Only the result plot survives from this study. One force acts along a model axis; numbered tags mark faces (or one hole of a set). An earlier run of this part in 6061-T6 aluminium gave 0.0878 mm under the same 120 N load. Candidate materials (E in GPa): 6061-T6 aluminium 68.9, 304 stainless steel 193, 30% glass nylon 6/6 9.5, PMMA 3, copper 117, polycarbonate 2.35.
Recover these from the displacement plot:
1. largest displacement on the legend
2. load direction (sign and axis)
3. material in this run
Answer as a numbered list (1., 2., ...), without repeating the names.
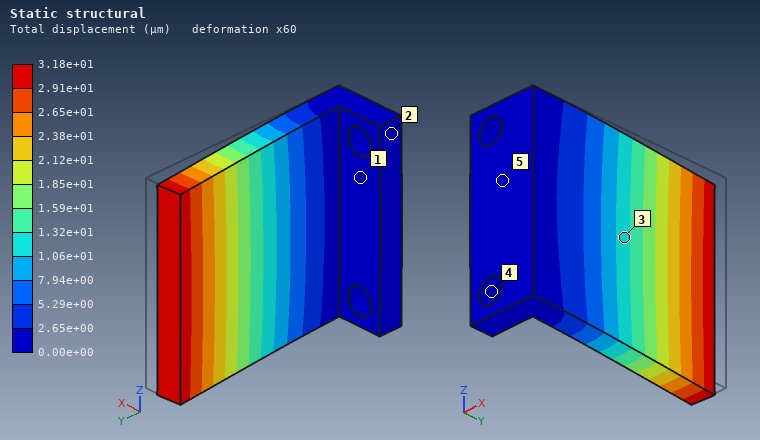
1. 3.18e+01 µm
2. -X
3. 304 stainless steel
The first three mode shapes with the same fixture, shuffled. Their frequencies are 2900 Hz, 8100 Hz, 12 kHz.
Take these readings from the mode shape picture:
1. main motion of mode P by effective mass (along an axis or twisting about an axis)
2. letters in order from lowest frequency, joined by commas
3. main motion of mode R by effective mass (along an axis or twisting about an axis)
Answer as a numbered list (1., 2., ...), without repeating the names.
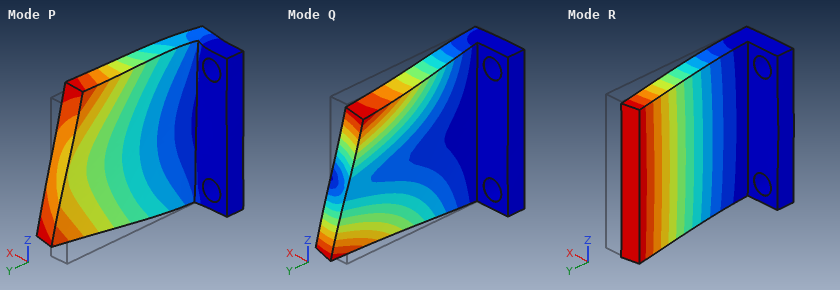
1. along Z
2. R, Q, P
3. along X
